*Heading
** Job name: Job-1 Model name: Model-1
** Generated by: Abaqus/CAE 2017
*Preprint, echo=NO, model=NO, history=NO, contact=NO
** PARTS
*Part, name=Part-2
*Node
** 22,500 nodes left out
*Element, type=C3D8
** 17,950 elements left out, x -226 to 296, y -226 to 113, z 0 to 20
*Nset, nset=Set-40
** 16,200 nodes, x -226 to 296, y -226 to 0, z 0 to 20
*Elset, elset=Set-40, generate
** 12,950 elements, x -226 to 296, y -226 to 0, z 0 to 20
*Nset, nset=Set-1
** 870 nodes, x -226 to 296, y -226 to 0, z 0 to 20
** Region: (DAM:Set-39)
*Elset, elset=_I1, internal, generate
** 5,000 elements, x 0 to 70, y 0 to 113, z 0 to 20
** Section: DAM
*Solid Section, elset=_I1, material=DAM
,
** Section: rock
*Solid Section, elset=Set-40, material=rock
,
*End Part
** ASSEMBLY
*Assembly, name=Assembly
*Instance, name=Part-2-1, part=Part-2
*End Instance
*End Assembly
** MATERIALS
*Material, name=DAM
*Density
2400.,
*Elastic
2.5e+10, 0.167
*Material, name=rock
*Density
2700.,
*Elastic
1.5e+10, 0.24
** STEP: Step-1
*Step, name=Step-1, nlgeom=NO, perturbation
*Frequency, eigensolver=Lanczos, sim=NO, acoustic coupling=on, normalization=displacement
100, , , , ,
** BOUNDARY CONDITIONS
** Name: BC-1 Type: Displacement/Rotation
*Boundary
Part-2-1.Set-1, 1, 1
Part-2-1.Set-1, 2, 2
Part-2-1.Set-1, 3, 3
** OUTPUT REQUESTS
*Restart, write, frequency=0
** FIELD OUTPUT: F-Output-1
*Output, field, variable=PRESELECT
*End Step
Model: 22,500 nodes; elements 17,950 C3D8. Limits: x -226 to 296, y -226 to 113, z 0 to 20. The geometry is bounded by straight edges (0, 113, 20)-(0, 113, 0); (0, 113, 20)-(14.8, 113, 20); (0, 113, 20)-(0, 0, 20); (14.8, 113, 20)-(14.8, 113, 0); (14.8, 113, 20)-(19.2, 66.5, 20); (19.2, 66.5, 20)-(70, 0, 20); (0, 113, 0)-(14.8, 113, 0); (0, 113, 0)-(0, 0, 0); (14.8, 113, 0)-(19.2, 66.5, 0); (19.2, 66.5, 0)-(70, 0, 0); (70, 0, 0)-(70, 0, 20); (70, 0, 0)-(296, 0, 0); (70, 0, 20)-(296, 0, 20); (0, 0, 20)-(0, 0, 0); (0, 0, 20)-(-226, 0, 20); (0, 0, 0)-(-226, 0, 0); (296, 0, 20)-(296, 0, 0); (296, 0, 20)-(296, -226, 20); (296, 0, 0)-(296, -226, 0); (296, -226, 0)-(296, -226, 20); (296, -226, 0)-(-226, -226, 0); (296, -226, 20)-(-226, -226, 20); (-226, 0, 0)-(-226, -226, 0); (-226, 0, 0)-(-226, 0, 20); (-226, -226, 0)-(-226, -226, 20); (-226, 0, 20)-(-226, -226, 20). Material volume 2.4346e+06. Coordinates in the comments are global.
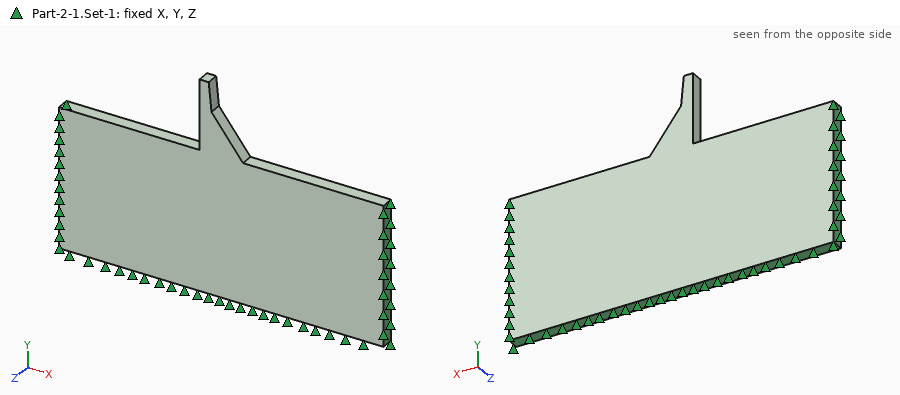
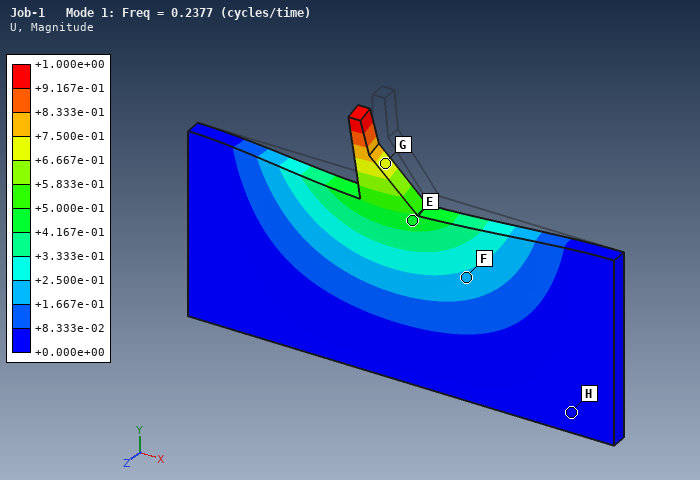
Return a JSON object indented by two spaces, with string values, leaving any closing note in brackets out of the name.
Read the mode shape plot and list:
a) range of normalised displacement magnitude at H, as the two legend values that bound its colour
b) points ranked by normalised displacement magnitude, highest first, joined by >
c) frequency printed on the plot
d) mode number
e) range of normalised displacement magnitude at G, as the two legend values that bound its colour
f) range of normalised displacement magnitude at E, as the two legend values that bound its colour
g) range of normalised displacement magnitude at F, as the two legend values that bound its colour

{
  "range of normalised displacement magnitude at H, as the two legend values that bound its colour": "+0.000e+00 to +8.333e-02",
  "points ranked by normalised displacement magnitude, highest first, joined by >": "G > E > F > H",
  "frequency printed on the plot": "0.2377",
  "mode number": "1",
  "range of normalised displacement magnitude at G, as the two legend values that bound its colour": "+6.667e-01 to +7.500e-01",
  "range of normalised displacement magnitude at E, as the two legend values that bound its colour": "+4.167e-01 to +5.000e-01",
  "range of normalised displacement magnitude at F, as the two legend values that bound its colour": "+1.667e-01 to +2.500e-01"
}
